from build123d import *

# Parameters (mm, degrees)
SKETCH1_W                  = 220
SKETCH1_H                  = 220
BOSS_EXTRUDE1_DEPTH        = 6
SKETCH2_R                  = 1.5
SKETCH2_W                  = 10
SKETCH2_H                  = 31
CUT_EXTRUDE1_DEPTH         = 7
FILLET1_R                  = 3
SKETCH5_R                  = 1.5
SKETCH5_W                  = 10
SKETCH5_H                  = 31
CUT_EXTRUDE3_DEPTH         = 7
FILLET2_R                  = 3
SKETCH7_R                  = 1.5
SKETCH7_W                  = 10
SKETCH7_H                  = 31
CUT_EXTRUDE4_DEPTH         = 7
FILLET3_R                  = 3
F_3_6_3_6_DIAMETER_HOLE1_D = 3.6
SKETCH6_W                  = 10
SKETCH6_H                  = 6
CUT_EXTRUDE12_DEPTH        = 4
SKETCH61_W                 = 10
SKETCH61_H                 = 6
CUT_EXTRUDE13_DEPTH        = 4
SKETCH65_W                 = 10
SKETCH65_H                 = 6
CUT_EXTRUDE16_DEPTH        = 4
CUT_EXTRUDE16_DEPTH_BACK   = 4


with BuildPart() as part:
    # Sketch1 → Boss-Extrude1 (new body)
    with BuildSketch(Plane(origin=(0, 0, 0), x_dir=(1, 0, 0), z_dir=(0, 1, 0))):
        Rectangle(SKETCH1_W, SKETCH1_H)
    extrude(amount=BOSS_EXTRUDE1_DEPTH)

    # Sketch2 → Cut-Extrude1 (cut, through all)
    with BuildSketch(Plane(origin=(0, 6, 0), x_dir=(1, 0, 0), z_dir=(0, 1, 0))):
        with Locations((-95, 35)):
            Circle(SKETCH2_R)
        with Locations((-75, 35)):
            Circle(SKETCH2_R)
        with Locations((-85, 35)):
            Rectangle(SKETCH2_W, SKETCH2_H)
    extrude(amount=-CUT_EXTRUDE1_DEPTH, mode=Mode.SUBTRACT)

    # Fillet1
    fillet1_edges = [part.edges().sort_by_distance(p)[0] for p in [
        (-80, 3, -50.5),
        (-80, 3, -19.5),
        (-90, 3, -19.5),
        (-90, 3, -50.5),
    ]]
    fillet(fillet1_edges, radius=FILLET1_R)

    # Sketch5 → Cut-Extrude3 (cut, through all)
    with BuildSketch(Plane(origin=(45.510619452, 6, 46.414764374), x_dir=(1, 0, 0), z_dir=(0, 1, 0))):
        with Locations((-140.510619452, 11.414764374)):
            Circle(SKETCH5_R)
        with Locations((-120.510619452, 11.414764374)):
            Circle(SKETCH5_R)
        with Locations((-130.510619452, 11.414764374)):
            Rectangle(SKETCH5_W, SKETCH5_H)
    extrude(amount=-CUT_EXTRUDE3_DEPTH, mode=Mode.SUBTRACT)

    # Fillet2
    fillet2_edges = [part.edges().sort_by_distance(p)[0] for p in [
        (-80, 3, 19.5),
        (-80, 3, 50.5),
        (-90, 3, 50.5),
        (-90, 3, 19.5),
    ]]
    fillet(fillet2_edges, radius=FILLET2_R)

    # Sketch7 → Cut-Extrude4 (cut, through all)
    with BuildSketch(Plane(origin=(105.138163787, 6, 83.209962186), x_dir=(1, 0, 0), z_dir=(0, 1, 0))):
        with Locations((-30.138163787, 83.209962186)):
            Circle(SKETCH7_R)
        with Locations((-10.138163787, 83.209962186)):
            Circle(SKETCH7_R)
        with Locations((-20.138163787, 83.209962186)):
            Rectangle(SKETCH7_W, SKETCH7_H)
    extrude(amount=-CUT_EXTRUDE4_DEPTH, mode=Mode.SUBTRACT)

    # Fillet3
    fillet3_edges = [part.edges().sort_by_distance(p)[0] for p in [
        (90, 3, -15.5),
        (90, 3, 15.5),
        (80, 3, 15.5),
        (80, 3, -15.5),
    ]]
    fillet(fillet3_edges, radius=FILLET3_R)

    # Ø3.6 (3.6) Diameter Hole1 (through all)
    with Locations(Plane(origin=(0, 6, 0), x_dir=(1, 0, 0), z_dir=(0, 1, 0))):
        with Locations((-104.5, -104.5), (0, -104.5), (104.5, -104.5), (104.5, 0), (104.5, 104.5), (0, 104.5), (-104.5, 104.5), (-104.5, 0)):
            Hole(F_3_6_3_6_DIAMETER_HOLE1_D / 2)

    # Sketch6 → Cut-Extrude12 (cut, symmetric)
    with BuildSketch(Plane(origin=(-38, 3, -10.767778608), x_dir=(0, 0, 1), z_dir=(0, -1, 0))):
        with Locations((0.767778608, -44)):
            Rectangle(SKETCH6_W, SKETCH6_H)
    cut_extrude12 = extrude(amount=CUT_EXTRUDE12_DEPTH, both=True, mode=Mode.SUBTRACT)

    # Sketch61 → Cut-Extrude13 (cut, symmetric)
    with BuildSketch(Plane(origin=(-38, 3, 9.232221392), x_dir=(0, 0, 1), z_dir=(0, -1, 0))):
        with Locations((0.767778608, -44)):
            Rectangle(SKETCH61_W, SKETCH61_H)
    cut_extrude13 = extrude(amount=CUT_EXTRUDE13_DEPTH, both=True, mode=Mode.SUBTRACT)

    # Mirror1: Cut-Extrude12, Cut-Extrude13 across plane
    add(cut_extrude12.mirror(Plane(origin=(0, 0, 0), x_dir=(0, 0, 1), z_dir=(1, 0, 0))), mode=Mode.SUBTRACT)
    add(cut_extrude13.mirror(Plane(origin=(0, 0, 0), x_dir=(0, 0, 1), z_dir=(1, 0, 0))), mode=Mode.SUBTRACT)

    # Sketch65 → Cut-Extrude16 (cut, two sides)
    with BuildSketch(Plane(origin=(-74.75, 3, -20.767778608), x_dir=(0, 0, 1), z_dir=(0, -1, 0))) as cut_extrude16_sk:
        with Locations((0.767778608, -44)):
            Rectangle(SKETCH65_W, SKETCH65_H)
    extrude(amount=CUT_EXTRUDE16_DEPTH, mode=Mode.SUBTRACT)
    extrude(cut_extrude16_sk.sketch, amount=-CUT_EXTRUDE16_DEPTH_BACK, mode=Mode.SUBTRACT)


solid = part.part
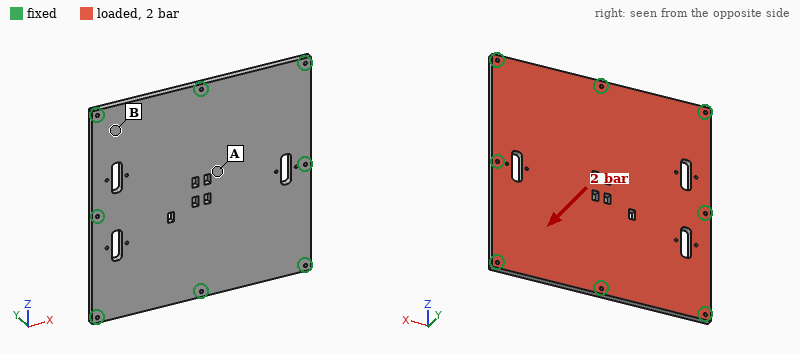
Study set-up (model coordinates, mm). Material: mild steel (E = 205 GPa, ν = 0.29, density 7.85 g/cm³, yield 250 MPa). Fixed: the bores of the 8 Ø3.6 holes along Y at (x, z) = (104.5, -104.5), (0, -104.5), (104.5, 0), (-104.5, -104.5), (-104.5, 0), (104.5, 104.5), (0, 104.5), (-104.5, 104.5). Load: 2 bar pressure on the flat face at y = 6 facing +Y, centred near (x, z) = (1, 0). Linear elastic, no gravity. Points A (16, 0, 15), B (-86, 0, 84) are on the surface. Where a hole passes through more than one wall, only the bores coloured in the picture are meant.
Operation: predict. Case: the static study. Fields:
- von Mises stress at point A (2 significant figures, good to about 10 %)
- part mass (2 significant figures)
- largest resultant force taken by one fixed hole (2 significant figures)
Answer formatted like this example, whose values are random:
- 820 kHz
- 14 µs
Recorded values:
- 44 MPa
- 2.2 kg
- 1.9 kN
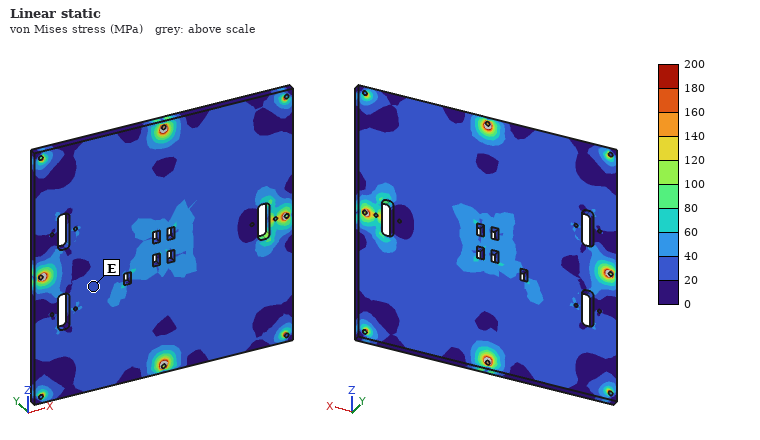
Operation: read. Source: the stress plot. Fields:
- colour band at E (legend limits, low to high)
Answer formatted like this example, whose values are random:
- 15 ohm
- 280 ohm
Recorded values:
- 20 to 40 MPa
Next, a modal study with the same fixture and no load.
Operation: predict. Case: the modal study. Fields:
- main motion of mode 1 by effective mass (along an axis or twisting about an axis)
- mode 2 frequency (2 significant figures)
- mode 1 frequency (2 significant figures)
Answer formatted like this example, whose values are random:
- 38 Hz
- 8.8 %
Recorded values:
- along Y
- 1600 Hz
- 870 Hz
